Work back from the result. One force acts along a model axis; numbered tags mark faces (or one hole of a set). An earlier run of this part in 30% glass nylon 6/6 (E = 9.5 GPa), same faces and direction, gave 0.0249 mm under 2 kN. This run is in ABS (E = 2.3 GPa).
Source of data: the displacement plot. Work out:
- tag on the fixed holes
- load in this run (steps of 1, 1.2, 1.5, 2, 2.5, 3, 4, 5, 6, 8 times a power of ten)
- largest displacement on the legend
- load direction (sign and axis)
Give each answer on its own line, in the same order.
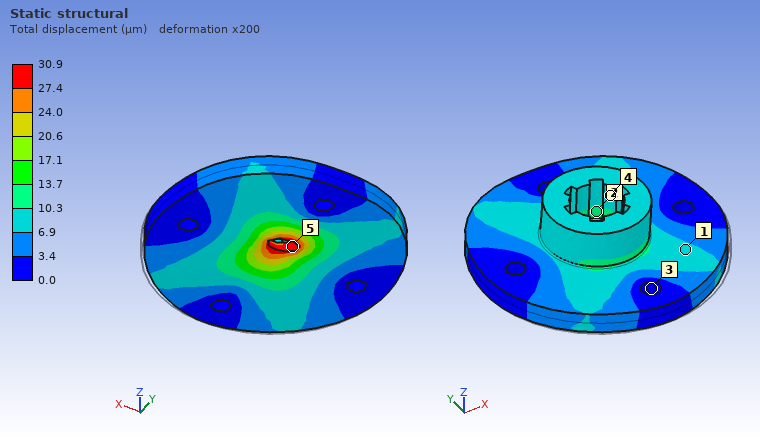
3
600 N
30.9 µm
+Y
